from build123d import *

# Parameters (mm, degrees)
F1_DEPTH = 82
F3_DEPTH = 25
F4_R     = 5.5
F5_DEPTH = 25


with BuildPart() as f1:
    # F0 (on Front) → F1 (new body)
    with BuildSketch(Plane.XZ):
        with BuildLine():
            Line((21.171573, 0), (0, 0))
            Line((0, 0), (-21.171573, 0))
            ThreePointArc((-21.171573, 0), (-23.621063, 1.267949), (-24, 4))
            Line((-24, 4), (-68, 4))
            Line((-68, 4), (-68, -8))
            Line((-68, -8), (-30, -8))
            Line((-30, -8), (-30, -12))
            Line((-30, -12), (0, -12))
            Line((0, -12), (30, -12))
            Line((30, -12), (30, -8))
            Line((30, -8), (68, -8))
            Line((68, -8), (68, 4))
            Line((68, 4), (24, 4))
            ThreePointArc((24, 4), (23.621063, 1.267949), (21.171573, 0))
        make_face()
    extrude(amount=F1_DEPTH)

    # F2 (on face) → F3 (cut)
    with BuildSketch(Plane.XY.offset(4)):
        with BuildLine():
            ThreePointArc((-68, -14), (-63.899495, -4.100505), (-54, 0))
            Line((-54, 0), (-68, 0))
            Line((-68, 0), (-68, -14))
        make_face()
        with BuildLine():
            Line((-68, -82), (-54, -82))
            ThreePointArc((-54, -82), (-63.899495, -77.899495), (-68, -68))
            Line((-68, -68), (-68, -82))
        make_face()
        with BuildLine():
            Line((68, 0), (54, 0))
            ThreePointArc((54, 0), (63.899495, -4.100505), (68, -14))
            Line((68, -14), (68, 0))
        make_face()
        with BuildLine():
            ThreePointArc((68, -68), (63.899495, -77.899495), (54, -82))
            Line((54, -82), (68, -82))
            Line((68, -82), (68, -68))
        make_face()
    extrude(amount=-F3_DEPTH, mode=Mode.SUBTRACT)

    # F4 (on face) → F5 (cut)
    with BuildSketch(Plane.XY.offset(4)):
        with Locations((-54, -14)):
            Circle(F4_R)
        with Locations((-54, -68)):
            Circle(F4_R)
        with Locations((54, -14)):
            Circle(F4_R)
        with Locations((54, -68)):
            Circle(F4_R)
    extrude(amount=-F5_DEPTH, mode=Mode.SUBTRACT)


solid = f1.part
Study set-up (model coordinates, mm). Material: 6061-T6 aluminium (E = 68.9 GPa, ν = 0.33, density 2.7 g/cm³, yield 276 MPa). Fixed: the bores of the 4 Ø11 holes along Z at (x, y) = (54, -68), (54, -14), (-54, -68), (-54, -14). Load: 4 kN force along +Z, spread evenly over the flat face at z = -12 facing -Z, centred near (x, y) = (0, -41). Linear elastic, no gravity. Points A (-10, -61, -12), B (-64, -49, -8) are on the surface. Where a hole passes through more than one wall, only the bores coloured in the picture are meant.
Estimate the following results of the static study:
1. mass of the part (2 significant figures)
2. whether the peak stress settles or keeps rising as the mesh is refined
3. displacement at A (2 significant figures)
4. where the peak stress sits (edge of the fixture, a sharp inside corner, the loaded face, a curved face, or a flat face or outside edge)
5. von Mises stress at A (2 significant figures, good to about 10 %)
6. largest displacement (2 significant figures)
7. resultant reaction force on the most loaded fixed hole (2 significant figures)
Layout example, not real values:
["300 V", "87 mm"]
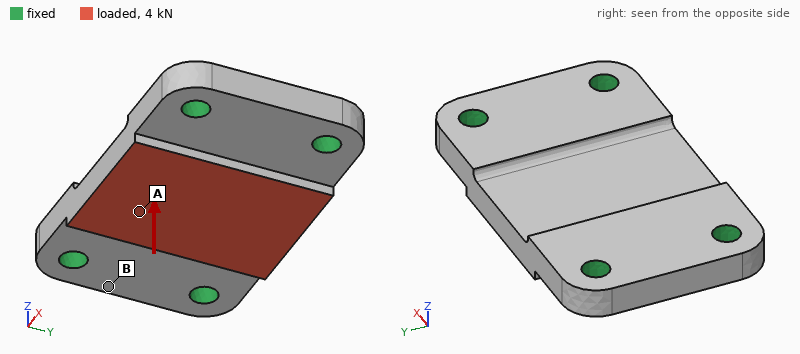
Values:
["350 g", "keeps rising", "21 µm", "edge of the fixture", "12 MPa", "23 µm", "1.6 kN"]
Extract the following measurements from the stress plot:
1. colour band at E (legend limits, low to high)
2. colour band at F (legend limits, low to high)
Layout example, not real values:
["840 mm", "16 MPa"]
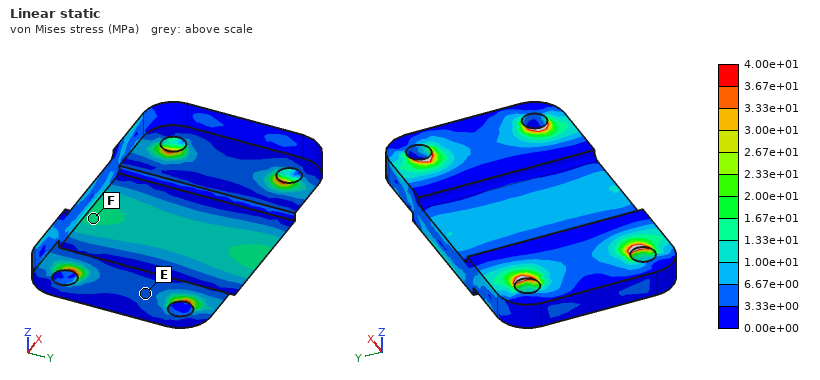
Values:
["3.33e+00 to 6.67e+00 MPa", "1.33e+01 to 1.67e+01 MPa"]
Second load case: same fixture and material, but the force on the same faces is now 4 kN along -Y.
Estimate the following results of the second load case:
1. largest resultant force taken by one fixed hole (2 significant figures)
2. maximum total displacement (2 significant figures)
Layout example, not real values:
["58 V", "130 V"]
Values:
["1.4 kN", "11 µm"]
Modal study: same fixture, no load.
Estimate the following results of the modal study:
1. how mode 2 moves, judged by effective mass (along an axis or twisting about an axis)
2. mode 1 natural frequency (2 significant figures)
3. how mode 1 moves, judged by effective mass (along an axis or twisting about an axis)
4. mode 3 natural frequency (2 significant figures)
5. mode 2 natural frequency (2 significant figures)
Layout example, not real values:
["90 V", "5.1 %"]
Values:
["twisting about X", "5400 Hz", "along Z", "12 kHz", "7000 Hz"]
